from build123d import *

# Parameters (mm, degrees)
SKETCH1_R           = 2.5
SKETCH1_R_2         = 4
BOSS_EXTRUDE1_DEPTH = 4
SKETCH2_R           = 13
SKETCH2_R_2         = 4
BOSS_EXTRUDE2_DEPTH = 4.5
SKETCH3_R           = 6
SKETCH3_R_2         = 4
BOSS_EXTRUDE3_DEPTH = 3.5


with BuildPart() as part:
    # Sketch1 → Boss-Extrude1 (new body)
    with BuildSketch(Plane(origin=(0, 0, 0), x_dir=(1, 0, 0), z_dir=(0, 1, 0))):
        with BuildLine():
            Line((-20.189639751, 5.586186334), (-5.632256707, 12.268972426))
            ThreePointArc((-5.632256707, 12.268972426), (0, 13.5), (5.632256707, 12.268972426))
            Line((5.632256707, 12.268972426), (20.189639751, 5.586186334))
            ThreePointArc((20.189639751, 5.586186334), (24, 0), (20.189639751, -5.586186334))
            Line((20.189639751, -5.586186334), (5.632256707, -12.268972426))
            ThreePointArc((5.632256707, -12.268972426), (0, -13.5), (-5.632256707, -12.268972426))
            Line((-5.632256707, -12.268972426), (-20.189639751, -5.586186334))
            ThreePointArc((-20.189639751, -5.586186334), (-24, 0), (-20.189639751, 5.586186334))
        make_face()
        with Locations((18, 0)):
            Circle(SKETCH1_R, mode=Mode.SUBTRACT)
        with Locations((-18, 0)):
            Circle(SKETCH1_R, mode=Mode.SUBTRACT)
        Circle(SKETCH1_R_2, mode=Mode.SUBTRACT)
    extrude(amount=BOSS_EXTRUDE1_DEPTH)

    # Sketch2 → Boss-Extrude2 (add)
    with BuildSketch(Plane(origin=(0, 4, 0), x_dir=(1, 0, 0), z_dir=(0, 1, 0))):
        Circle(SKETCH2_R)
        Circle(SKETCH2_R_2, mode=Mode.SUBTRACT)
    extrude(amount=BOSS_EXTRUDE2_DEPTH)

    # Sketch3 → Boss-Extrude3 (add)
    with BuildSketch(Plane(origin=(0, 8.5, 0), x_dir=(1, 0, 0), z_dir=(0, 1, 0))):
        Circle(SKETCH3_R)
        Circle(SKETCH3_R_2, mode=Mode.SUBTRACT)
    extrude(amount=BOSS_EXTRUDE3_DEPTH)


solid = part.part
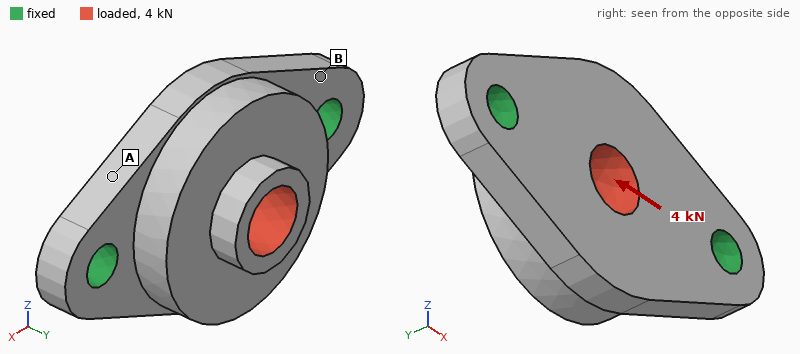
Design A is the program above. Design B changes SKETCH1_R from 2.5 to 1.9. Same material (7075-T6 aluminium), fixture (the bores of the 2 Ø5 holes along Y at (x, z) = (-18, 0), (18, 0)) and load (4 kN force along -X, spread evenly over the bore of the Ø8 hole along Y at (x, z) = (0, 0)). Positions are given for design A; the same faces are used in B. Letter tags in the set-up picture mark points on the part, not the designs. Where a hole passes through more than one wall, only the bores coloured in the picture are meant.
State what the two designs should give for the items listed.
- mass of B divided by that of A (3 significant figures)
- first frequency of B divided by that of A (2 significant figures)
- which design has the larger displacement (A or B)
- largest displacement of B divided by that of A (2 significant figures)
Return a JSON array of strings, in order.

["1.01", "0.89", "B", "1.1"]
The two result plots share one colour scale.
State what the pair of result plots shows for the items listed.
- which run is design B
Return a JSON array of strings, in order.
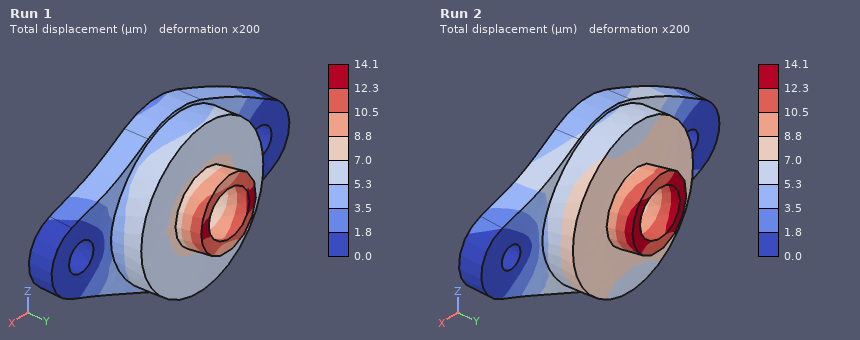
["Run 2"]
